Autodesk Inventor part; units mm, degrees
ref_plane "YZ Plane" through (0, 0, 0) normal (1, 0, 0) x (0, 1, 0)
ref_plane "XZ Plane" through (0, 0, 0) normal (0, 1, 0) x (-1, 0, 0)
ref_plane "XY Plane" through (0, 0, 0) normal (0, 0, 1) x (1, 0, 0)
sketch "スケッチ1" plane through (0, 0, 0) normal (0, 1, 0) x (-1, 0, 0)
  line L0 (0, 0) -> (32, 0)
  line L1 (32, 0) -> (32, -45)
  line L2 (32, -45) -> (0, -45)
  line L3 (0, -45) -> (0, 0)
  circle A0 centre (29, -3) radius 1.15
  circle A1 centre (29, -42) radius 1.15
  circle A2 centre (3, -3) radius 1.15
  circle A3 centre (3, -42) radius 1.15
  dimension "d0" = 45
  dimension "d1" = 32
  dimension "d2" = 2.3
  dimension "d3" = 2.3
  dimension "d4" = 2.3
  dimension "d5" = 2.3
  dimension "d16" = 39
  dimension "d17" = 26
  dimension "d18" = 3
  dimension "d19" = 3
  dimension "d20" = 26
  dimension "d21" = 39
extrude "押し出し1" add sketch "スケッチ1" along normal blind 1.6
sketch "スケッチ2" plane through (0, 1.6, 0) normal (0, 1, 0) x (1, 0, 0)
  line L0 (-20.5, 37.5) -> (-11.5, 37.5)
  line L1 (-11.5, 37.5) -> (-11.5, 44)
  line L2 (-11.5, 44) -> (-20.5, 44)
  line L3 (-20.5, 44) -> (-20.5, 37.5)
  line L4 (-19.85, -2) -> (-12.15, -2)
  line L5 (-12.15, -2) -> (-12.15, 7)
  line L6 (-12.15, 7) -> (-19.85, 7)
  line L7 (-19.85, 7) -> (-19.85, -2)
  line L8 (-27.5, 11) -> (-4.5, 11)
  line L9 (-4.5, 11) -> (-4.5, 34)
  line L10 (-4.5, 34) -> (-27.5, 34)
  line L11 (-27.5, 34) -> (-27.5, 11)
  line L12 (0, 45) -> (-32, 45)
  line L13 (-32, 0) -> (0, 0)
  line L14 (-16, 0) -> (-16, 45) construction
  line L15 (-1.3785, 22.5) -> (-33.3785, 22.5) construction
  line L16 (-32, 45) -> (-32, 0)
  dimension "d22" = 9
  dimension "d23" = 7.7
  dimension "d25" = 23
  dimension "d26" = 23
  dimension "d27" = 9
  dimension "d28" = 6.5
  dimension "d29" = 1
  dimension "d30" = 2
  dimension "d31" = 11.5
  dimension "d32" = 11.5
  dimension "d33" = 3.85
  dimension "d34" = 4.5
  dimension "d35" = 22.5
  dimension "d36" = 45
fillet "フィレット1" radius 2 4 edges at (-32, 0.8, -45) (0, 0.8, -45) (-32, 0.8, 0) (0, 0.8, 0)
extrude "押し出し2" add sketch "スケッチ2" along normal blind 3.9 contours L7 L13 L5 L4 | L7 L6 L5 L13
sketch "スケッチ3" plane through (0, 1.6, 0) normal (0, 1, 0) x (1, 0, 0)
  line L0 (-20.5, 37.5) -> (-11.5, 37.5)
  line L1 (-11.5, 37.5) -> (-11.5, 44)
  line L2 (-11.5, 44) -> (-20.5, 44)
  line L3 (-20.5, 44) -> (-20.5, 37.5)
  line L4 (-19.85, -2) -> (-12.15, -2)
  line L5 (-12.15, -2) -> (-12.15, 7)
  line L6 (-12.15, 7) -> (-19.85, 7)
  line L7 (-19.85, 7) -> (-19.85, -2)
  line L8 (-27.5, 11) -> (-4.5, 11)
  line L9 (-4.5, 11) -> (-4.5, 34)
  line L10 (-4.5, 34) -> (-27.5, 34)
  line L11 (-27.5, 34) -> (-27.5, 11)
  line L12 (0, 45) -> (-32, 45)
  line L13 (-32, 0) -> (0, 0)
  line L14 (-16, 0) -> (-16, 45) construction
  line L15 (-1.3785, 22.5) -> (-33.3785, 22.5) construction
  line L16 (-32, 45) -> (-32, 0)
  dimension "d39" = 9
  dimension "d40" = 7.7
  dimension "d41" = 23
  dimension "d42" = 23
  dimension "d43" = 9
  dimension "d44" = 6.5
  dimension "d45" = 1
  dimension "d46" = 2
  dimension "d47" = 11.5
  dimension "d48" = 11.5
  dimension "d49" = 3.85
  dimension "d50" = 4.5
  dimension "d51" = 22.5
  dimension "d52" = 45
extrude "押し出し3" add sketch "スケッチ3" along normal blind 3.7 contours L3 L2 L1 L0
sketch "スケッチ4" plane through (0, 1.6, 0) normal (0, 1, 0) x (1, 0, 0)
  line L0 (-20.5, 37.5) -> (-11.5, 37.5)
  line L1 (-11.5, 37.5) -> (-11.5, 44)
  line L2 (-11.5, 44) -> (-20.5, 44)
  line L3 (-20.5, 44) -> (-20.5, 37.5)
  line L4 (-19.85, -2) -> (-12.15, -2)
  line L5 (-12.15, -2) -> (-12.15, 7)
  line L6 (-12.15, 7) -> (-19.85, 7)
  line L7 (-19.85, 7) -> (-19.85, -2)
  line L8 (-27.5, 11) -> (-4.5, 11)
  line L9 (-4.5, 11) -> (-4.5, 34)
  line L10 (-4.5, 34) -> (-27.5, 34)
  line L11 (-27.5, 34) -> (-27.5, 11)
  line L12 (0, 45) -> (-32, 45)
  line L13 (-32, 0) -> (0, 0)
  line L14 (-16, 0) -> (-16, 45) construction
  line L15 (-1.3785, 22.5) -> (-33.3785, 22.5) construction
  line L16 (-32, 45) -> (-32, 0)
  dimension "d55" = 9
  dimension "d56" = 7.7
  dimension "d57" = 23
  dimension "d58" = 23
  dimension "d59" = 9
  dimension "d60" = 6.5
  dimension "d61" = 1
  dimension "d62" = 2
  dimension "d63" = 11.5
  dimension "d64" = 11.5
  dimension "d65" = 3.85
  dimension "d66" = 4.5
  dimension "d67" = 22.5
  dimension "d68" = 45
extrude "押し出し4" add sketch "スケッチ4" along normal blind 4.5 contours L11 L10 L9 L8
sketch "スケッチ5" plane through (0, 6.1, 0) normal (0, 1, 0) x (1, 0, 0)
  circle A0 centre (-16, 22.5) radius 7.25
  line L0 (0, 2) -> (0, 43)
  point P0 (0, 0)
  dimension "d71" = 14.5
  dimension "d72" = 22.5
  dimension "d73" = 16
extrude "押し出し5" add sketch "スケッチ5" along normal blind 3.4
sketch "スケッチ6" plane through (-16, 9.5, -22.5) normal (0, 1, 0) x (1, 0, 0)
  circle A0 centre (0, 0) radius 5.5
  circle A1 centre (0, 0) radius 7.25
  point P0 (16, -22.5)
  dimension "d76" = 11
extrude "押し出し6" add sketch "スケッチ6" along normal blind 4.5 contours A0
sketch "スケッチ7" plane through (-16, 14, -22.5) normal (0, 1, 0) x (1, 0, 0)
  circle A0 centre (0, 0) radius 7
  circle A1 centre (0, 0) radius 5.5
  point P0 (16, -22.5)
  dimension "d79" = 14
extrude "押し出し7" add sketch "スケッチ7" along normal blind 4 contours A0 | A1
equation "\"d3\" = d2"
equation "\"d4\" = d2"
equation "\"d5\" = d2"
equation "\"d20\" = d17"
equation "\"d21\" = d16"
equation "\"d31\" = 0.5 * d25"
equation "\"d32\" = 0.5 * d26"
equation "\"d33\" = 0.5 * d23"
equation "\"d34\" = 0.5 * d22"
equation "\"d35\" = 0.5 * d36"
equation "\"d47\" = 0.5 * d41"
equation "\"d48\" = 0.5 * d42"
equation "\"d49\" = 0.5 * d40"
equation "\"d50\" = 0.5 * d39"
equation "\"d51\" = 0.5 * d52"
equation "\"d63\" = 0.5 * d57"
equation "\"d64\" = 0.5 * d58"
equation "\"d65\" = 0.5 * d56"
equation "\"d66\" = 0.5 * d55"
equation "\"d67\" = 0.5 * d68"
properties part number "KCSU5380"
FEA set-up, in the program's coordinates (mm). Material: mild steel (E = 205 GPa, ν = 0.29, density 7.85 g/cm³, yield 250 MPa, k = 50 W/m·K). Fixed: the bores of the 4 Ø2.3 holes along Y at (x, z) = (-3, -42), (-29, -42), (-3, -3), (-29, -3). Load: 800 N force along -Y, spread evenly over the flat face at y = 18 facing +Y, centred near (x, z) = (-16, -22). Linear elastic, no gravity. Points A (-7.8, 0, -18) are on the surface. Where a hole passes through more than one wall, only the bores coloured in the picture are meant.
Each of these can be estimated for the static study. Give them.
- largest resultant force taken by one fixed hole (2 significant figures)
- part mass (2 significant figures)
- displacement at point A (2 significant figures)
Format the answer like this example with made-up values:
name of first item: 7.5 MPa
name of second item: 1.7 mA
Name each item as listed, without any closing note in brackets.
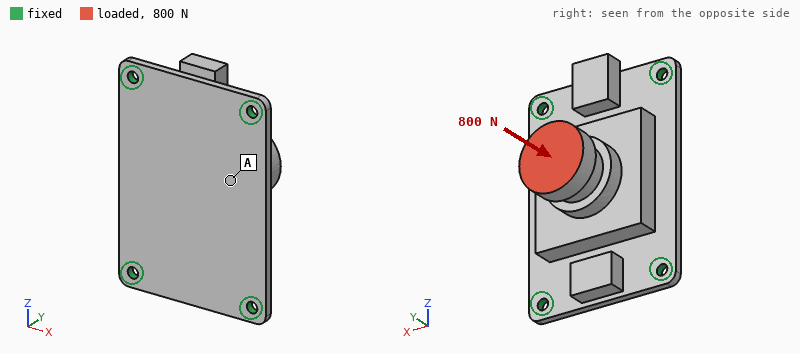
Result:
largest resultant force taken by one fixed hole: 260 N
part mass: 53 g
displacement at point A: 22 µm
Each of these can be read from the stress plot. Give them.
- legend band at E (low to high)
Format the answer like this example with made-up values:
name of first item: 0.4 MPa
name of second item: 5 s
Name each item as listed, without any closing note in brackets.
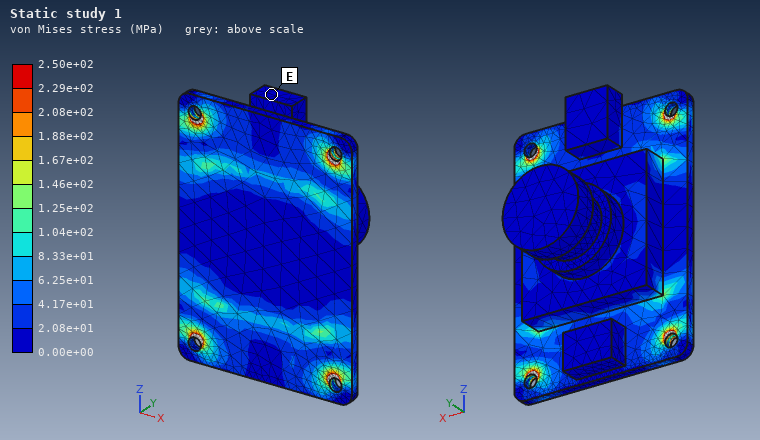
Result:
legend band at E: 0.00e+00 to 2.08e+01 MPa
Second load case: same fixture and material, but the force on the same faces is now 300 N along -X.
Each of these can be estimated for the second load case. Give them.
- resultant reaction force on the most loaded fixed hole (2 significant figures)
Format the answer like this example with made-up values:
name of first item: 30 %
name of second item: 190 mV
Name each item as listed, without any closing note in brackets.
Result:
resultant reaction force on the most loaded fixed hole: 160 N
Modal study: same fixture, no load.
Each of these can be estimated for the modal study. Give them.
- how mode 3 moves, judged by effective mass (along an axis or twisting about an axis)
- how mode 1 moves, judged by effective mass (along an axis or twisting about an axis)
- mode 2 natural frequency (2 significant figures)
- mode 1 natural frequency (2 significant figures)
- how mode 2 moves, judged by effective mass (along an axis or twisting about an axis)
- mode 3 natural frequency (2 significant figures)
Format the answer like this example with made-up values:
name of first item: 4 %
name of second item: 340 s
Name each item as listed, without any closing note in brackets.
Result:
how mode 3 moves, judged by effective mass: along Z
how mode 1 moves, judged by effective mass: along Y
mode 2 natural frequency: 5900 Hz
mode 1 natural frequency: 4700 Hz
how mode 2 moves, judged by effective mass: along X
mode 3 natural frequency: 7700 Hz
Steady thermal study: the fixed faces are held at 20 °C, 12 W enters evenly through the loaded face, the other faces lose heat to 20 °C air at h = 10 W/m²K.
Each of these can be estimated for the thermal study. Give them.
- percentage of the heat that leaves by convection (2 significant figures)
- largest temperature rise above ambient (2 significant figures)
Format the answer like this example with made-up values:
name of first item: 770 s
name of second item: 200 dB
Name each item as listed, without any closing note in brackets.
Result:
percentage of the heat that leaves by convection: 9.7 %
largest temperature rise above ambient: 63 K
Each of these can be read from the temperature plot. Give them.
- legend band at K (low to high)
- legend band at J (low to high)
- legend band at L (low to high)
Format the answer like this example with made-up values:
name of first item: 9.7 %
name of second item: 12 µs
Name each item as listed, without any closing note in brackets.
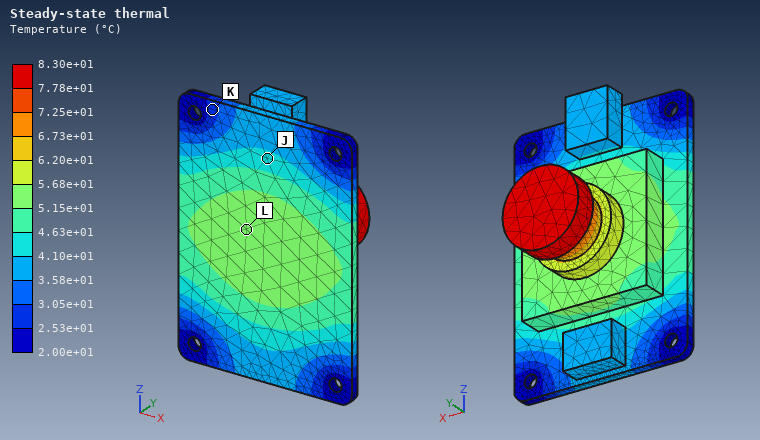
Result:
legend band at K: 2.53e+01 to 3.05e+01 °C
legend band at J: 4.10e+01 to 4.63e+01 °C
legend band at L: 5.15e+01 to 5.68e+01 °C
